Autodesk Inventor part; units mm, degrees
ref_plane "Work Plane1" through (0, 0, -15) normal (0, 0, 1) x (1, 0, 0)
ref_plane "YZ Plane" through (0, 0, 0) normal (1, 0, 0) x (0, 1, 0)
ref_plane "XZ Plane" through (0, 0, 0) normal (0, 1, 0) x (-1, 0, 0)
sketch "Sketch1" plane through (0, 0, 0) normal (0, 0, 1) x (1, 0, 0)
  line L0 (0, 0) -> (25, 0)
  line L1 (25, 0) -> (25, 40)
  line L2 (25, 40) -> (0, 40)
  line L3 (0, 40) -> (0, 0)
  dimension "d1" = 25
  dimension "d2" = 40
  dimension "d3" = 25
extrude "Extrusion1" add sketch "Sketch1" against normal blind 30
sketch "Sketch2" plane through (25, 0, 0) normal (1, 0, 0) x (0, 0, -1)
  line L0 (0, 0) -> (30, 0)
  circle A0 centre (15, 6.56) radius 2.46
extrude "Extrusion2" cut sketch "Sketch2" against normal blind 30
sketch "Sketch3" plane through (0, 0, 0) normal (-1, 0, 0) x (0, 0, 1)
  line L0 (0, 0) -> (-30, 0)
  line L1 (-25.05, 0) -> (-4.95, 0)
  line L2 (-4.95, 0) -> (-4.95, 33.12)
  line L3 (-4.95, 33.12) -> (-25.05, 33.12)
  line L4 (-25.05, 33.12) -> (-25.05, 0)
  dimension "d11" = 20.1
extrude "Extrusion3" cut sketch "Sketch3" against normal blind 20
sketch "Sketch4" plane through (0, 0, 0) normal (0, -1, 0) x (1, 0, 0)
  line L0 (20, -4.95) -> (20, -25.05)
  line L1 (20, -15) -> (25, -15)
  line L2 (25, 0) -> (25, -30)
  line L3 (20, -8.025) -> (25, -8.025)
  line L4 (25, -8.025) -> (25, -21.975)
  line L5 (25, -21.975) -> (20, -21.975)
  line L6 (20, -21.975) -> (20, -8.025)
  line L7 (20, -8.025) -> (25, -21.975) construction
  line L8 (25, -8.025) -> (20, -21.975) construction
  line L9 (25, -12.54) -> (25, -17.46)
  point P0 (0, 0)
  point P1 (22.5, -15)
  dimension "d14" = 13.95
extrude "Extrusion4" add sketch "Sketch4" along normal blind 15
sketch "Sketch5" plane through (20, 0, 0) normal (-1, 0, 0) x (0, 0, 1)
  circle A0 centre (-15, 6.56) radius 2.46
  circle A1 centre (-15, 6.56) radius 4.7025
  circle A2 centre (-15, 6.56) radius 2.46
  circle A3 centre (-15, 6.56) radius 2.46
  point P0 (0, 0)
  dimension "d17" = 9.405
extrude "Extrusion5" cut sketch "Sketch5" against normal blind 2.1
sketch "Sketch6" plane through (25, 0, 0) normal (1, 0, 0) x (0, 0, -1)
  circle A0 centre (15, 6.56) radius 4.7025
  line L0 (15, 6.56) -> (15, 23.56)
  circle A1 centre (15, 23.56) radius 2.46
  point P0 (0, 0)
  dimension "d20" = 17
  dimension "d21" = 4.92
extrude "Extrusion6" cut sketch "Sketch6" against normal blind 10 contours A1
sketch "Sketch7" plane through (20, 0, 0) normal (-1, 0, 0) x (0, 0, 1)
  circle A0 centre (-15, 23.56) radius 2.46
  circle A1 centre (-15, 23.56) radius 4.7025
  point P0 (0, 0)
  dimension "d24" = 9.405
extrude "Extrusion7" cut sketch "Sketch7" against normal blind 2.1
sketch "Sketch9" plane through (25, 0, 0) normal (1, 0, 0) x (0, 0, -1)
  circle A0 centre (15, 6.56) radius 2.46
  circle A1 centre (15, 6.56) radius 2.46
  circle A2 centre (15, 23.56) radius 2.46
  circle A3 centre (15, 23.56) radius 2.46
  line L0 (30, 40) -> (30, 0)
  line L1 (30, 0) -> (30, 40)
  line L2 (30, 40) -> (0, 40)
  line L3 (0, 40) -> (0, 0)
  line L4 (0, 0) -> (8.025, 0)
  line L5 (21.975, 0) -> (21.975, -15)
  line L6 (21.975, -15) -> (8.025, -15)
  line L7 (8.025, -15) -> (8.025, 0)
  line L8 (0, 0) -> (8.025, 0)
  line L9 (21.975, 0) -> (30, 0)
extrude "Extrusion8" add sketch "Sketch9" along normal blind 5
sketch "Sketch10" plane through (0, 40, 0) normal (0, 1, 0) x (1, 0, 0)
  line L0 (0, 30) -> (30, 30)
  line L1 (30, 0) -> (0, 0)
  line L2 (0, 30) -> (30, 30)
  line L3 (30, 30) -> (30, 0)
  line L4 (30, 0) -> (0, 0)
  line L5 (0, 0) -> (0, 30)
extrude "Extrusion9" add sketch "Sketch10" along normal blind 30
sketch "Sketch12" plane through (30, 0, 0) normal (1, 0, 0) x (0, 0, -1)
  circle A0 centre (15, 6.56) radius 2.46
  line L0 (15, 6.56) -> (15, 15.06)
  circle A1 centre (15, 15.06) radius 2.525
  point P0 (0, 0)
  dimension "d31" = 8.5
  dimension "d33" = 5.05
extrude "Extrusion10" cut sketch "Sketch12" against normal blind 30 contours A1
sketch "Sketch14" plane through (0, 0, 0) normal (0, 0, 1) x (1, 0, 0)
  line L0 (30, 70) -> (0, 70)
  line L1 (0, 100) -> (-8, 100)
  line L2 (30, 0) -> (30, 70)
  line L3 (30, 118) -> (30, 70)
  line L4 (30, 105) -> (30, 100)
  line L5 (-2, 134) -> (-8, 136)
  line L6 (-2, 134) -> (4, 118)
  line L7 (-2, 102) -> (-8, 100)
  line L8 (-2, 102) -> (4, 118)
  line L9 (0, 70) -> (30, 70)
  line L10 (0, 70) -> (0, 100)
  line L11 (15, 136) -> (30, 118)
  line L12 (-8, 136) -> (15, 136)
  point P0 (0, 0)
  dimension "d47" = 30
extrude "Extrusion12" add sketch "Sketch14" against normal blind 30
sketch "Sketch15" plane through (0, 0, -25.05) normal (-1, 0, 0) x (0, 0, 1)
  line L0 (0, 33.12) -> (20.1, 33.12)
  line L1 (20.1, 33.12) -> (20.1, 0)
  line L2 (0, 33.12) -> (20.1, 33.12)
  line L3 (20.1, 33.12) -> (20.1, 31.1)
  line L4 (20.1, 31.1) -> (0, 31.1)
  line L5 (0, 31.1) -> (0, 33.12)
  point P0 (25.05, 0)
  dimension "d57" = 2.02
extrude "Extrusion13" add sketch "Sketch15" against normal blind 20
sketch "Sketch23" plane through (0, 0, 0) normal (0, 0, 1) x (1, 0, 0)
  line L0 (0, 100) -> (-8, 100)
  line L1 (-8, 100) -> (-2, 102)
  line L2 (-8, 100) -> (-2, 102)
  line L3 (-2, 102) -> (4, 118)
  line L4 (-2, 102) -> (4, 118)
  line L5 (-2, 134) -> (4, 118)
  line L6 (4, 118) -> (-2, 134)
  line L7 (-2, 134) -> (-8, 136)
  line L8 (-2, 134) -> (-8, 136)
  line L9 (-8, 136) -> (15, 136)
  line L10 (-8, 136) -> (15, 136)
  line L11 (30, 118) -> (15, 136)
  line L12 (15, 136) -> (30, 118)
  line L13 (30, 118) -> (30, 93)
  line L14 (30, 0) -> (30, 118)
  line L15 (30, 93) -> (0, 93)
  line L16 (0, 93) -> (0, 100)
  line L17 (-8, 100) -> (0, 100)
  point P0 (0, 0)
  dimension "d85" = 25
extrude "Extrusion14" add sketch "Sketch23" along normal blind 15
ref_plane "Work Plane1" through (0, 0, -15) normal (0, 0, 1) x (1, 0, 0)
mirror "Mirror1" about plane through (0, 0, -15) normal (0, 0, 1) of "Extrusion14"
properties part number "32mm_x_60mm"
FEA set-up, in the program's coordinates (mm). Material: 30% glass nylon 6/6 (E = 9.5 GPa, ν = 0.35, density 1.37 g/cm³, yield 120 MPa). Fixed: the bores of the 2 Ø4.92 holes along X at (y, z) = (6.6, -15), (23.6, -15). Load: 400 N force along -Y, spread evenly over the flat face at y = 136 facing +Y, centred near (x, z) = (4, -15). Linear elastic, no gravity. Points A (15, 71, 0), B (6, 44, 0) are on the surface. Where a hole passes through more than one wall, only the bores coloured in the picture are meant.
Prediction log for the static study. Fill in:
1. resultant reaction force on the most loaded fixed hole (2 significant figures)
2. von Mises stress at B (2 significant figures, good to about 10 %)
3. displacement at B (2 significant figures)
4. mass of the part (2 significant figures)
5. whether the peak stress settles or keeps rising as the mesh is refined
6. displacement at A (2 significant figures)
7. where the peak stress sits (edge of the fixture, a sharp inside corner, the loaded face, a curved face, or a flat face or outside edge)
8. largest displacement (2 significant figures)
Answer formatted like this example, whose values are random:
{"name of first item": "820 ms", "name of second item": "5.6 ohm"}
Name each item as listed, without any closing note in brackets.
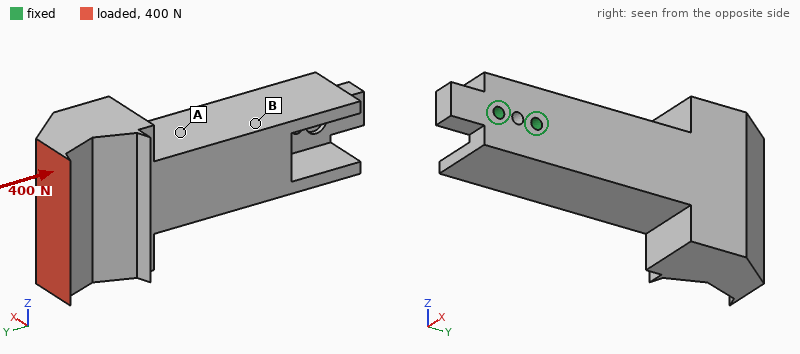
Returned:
{"resultant reaction force on the most loaded fixed hole": "410 N", "von Mises stress at B": "1.7 MPa", "displacement at B": "0.042 mm", "mass of the part": "190 g", "whether the peak stress settles or keeps rising as the mesh is refined": "keeps rising", "displacement at A": "0.074 mm", "where the peak stress sits": "edge of the fixture", "largest displacement": "0.22 mm"}
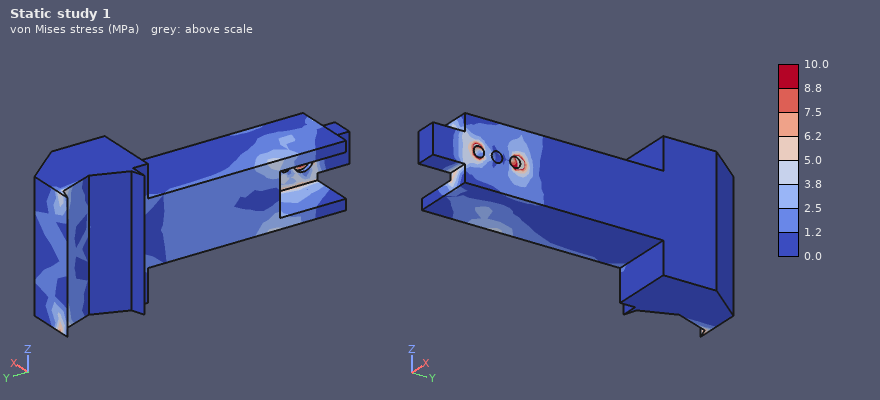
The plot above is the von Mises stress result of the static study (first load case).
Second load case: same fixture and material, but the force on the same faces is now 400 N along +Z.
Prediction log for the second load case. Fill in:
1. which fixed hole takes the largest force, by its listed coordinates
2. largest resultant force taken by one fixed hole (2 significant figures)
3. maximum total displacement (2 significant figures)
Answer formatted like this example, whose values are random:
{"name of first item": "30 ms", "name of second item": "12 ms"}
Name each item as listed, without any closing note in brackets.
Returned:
{"which fixed hole takes the largest force, by its listed coordinates": "(23.6, -15)", "largest resultant force taken by one fixed hole": "2.3 kN", "maximum total displacement": "0.89 mm"}
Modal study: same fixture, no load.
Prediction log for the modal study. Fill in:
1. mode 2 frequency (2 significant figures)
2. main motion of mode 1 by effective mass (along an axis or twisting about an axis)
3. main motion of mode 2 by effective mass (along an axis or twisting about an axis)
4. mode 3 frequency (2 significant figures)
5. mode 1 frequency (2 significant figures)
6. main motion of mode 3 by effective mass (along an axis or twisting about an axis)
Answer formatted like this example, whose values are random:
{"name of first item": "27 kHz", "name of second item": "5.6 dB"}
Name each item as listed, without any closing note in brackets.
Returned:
{"mode 2 frequency": "430 Hz", "main motion of mode 1 by effective mass": "along X", "main motion of mode 2 by effective mass": "along Z", "mode 3 frequency": "1000 Hz", "mode 1 frequency": "370 Hz", "main motion of mode 3 by effective mass": "twisting about Y"}
